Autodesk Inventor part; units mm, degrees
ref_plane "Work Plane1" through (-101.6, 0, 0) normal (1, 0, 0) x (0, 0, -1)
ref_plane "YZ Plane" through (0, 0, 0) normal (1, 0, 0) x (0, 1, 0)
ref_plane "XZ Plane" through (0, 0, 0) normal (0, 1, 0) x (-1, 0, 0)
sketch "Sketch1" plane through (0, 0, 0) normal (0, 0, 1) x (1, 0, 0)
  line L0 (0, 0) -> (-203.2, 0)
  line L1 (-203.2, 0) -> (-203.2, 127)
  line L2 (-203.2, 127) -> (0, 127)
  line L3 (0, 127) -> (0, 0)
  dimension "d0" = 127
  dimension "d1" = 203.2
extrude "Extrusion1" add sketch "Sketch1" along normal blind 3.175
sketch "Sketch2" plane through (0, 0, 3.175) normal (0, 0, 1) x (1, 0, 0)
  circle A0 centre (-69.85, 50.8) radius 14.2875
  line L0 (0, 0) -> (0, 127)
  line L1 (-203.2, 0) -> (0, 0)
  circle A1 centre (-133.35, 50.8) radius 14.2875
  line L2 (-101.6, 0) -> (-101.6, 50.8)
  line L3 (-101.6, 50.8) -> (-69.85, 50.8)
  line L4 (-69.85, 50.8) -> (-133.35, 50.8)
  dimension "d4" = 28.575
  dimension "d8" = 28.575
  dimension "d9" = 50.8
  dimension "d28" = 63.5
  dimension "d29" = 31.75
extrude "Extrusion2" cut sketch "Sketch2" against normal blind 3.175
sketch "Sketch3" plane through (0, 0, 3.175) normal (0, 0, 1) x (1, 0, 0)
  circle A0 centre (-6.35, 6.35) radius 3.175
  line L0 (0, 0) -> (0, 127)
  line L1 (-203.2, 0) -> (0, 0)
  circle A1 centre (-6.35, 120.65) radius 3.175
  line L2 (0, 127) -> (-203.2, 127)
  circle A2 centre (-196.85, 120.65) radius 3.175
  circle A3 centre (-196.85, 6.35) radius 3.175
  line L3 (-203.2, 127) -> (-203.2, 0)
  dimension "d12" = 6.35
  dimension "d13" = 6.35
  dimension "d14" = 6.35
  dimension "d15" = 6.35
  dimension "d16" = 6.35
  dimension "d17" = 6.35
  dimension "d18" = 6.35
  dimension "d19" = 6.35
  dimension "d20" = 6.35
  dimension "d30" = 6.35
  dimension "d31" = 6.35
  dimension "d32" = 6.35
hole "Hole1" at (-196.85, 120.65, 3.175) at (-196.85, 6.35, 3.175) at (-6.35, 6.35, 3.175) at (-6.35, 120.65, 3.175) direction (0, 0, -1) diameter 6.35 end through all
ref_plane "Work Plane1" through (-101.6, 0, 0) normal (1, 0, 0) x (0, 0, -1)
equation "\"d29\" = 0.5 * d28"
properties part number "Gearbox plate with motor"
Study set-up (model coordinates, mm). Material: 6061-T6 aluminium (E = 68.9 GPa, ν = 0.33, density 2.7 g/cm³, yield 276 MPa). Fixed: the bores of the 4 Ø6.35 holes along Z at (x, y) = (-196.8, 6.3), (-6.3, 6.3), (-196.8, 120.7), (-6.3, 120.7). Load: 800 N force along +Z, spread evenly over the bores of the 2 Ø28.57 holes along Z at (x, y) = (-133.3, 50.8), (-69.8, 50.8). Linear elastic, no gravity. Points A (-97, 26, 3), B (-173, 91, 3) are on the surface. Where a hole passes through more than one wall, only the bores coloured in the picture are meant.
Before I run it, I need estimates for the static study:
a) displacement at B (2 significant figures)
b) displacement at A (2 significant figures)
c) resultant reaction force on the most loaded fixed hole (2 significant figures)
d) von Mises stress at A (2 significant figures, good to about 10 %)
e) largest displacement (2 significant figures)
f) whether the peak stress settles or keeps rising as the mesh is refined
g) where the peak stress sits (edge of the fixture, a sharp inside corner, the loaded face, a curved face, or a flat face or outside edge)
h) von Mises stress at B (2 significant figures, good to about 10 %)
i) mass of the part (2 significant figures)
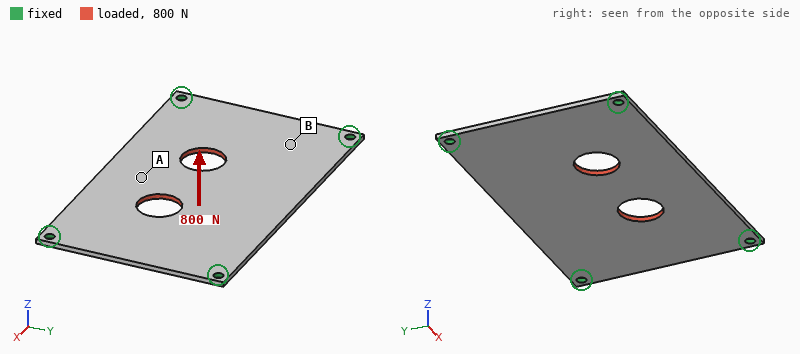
0.46 mm
1.7 mm
250 N
54 MPa
1.8 mm
keeps rising
edge of the fixture
27 MPa
210 g
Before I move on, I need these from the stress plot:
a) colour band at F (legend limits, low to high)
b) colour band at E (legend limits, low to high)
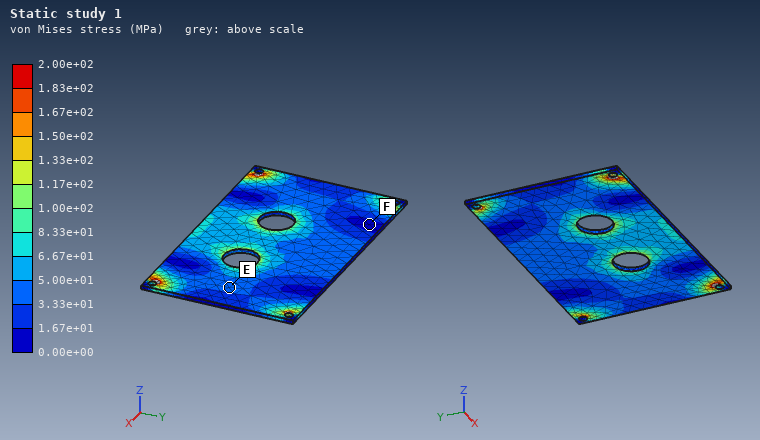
0.00e+00 to 1.67e+01 MPa
3.33e+01 to 5.00e+01 MPa
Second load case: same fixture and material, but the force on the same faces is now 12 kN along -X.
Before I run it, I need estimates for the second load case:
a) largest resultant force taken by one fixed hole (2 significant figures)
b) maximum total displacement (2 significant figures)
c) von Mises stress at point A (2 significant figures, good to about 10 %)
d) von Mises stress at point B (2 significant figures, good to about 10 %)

3.5 kN
47 µm
18 MPa
21 MPa
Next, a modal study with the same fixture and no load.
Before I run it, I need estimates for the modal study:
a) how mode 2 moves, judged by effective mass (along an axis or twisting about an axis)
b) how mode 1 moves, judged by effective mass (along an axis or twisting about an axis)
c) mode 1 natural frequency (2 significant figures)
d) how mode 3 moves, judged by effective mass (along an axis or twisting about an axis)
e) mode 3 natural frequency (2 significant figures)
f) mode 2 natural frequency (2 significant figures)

twisting about X
along Z
370 Hz
twisting about Y
950 Hz
630 Hz
